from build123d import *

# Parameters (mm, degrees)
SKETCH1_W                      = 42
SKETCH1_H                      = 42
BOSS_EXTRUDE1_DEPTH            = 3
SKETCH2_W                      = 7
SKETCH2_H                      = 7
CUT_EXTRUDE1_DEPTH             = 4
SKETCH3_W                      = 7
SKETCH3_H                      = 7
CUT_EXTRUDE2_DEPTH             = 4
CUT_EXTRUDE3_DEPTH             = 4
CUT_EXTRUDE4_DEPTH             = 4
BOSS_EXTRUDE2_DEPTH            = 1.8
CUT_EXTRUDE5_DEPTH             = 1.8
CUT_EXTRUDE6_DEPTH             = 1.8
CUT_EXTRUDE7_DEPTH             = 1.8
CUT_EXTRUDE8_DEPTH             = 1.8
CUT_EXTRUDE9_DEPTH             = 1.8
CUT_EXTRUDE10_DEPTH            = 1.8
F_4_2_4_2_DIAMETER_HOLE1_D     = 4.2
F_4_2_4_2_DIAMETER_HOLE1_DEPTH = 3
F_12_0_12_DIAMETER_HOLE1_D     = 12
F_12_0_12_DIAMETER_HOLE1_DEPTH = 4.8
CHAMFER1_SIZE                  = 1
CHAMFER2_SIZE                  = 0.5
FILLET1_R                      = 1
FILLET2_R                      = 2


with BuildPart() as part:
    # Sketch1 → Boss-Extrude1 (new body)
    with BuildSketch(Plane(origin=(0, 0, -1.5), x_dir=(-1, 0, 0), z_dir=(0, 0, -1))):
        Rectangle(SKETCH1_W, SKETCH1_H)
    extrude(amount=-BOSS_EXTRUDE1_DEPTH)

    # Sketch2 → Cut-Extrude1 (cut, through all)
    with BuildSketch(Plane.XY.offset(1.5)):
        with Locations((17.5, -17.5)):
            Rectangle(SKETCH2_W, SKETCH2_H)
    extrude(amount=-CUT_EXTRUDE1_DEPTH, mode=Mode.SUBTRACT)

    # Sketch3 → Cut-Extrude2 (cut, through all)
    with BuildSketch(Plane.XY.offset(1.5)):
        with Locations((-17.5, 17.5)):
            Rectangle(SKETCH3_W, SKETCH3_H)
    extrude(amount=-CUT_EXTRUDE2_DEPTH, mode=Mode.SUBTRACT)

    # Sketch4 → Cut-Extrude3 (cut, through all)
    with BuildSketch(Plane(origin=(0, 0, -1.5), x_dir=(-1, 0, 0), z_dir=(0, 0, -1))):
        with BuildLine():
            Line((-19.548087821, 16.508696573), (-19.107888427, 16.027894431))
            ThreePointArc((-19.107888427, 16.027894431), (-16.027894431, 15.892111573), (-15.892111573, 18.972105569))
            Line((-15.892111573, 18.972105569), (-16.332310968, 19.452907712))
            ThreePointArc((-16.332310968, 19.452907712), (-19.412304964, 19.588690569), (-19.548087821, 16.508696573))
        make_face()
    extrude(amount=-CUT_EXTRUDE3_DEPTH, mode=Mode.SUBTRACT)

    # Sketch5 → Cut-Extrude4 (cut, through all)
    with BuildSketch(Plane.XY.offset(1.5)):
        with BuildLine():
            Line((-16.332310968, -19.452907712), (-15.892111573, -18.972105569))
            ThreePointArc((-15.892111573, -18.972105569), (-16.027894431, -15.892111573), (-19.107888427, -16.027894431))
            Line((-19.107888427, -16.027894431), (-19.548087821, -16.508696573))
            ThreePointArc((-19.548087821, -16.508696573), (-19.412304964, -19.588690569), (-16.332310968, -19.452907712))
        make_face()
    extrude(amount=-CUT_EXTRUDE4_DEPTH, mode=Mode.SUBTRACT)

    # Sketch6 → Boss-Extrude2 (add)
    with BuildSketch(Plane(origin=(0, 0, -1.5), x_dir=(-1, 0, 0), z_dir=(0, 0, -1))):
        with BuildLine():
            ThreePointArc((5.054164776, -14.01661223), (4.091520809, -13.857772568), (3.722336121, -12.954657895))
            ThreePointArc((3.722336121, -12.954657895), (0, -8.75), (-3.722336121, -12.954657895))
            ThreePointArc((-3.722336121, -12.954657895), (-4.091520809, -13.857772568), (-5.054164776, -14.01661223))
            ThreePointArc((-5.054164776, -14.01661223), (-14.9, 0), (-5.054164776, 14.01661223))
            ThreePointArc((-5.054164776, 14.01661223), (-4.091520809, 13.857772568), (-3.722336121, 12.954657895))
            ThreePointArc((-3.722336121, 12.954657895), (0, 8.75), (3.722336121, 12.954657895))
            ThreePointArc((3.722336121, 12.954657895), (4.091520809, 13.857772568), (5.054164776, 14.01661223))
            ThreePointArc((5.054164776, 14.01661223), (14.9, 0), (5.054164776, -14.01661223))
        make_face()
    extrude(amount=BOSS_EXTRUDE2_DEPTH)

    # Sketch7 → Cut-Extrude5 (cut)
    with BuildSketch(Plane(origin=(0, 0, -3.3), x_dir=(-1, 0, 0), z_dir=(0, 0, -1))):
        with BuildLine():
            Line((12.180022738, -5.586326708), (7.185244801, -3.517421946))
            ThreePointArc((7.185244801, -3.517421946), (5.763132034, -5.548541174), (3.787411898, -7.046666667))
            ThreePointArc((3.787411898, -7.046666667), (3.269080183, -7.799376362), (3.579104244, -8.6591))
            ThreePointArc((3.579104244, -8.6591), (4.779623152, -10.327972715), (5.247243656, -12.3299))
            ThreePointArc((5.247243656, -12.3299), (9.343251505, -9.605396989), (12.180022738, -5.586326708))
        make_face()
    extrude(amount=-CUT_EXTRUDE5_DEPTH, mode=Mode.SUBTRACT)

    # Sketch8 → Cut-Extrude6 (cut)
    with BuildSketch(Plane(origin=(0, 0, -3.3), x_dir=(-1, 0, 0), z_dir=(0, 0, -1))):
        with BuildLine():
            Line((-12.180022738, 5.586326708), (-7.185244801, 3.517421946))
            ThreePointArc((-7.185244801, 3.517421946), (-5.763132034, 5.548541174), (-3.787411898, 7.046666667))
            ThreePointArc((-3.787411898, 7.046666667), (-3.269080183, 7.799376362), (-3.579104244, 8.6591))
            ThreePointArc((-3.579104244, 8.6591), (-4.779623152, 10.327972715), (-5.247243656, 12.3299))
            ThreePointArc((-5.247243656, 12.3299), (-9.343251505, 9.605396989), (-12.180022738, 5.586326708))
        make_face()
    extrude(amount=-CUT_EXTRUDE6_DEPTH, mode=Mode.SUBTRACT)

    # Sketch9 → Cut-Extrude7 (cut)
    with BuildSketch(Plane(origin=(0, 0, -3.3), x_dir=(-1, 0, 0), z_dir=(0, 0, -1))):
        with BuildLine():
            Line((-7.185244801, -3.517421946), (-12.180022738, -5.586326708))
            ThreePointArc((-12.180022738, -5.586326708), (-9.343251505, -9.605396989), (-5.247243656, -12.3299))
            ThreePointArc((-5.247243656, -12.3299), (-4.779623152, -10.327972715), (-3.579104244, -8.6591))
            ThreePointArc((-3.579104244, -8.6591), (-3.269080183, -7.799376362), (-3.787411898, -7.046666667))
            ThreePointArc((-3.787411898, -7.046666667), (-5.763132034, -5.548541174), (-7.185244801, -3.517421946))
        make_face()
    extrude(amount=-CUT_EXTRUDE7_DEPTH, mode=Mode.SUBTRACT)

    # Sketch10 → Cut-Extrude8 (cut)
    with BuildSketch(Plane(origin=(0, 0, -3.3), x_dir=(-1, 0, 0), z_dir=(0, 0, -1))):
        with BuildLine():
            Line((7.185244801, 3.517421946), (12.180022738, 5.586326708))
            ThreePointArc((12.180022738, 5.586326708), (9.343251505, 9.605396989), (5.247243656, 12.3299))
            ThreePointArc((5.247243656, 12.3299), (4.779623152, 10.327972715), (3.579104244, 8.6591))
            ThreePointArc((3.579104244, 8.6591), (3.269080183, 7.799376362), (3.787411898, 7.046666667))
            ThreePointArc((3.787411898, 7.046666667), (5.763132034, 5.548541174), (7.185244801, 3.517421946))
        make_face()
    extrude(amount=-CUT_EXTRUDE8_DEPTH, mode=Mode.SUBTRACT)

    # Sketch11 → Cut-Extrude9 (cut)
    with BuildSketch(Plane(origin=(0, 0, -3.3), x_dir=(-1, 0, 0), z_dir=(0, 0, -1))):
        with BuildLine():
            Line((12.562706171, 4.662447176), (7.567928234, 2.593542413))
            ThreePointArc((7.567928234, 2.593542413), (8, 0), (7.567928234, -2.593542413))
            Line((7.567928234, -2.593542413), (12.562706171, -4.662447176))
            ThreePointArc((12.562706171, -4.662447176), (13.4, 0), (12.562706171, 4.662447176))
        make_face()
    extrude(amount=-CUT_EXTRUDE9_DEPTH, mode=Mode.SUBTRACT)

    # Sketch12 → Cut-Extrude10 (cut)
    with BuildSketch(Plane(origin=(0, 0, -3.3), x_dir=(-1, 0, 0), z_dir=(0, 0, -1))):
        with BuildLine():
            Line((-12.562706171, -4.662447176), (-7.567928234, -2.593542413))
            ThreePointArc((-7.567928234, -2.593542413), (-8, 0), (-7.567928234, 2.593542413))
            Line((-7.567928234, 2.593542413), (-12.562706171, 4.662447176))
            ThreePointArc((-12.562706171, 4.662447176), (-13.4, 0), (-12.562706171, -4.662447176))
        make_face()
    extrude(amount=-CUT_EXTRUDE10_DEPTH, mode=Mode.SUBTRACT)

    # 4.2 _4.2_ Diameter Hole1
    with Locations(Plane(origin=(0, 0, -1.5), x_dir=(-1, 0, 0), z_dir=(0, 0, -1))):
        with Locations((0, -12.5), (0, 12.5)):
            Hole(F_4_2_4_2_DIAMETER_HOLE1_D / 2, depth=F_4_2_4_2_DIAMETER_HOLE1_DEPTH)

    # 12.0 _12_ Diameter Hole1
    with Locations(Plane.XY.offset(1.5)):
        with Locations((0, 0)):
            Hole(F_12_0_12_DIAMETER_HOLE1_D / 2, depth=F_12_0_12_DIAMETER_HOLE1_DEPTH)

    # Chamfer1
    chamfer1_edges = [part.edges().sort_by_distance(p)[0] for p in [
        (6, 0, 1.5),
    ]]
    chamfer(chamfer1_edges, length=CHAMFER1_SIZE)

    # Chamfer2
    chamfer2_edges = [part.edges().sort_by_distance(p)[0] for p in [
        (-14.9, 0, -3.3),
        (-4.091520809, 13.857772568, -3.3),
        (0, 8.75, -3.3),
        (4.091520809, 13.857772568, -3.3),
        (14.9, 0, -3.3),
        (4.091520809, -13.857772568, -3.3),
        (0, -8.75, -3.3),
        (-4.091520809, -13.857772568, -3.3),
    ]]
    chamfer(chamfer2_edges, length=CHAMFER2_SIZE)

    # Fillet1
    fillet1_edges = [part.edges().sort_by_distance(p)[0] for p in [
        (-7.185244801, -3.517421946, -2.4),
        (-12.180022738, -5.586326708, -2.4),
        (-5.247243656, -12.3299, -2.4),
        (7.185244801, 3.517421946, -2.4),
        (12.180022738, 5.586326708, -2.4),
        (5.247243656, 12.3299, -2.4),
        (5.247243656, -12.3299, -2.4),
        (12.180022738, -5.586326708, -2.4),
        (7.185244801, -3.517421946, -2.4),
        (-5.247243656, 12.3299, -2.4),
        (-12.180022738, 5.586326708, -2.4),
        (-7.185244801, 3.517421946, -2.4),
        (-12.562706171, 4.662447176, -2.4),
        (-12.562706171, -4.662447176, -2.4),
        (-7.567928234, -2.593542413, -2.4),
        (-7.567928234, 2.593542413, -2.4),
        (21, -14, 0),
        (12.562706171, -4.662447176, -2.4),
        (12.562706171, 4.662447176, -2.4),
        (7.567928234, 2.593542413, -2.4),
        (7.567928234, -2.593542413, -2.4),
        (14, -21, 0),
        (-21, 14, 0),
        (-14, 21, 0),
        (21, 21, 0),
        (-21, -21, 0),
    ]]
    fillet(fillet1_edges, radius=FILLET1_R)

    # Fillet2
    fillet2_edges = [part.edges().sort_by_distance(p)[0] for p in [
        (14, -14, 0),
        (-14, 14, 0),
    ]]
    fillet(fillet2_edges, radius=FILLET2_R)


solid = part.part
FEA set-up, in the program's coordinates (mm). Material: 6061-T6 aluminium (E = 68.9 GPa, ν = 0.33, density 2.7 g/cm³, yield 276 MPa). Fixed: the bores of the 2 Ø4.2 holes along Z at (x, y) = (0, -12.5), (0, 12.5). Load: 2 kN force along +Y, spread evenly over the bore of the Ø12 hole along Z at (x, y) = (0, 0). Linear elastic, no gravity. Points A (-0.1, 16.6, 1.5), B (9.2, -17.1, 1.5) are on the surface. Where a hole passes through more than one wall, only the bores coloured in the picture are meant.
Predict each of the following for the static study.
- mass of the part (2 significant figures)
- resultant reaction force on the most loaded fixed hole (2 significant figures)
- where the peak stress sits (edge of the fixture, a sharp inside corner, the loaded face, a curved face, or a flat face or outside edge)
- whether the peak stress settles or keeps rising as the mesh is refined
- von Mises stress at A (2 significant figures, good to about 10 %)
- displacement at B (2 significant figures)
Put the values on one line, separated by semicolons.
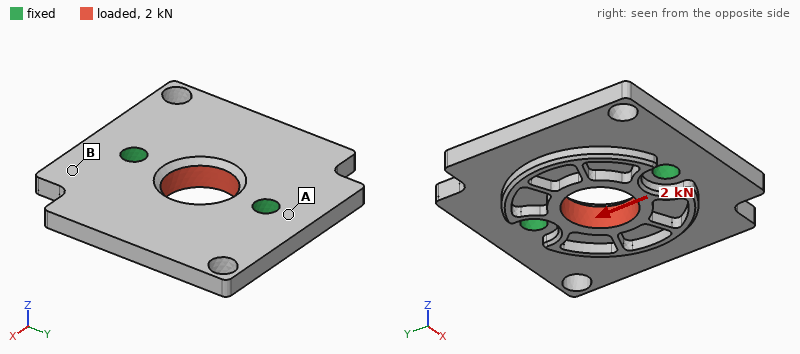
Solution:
13 g; 1.0 kN; edge of the fixture; keeps rising; 11 MPa; 2.3 µm
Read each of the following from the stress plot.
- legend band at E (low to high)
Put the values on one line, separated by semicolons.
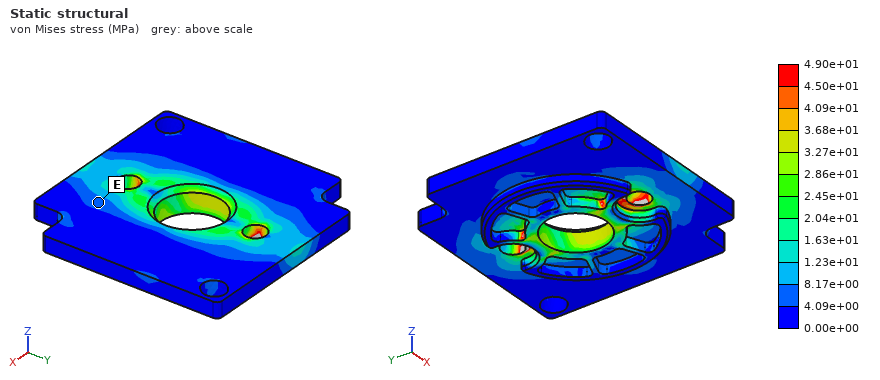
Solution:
4.09e+00 to 8.17e+00 MPa
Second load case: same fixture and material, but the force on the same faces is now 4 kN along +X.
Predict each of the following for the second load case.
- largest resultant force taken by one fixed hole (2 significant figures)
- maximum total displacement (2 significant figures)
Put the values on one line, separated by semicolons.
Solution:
2.0 kN; 49 µm
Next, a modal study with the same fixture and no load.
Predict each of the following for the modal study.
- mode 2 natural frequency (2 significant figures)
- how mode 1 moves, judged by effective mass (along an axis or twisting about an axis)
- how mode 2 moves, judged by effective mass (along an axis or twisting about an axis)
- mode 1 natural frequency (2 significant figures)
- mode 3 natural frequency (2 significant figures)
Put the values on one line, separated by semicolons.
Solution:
6700 Hz; twisting about Y; along Z; 5800 Hz; 11 kHz
